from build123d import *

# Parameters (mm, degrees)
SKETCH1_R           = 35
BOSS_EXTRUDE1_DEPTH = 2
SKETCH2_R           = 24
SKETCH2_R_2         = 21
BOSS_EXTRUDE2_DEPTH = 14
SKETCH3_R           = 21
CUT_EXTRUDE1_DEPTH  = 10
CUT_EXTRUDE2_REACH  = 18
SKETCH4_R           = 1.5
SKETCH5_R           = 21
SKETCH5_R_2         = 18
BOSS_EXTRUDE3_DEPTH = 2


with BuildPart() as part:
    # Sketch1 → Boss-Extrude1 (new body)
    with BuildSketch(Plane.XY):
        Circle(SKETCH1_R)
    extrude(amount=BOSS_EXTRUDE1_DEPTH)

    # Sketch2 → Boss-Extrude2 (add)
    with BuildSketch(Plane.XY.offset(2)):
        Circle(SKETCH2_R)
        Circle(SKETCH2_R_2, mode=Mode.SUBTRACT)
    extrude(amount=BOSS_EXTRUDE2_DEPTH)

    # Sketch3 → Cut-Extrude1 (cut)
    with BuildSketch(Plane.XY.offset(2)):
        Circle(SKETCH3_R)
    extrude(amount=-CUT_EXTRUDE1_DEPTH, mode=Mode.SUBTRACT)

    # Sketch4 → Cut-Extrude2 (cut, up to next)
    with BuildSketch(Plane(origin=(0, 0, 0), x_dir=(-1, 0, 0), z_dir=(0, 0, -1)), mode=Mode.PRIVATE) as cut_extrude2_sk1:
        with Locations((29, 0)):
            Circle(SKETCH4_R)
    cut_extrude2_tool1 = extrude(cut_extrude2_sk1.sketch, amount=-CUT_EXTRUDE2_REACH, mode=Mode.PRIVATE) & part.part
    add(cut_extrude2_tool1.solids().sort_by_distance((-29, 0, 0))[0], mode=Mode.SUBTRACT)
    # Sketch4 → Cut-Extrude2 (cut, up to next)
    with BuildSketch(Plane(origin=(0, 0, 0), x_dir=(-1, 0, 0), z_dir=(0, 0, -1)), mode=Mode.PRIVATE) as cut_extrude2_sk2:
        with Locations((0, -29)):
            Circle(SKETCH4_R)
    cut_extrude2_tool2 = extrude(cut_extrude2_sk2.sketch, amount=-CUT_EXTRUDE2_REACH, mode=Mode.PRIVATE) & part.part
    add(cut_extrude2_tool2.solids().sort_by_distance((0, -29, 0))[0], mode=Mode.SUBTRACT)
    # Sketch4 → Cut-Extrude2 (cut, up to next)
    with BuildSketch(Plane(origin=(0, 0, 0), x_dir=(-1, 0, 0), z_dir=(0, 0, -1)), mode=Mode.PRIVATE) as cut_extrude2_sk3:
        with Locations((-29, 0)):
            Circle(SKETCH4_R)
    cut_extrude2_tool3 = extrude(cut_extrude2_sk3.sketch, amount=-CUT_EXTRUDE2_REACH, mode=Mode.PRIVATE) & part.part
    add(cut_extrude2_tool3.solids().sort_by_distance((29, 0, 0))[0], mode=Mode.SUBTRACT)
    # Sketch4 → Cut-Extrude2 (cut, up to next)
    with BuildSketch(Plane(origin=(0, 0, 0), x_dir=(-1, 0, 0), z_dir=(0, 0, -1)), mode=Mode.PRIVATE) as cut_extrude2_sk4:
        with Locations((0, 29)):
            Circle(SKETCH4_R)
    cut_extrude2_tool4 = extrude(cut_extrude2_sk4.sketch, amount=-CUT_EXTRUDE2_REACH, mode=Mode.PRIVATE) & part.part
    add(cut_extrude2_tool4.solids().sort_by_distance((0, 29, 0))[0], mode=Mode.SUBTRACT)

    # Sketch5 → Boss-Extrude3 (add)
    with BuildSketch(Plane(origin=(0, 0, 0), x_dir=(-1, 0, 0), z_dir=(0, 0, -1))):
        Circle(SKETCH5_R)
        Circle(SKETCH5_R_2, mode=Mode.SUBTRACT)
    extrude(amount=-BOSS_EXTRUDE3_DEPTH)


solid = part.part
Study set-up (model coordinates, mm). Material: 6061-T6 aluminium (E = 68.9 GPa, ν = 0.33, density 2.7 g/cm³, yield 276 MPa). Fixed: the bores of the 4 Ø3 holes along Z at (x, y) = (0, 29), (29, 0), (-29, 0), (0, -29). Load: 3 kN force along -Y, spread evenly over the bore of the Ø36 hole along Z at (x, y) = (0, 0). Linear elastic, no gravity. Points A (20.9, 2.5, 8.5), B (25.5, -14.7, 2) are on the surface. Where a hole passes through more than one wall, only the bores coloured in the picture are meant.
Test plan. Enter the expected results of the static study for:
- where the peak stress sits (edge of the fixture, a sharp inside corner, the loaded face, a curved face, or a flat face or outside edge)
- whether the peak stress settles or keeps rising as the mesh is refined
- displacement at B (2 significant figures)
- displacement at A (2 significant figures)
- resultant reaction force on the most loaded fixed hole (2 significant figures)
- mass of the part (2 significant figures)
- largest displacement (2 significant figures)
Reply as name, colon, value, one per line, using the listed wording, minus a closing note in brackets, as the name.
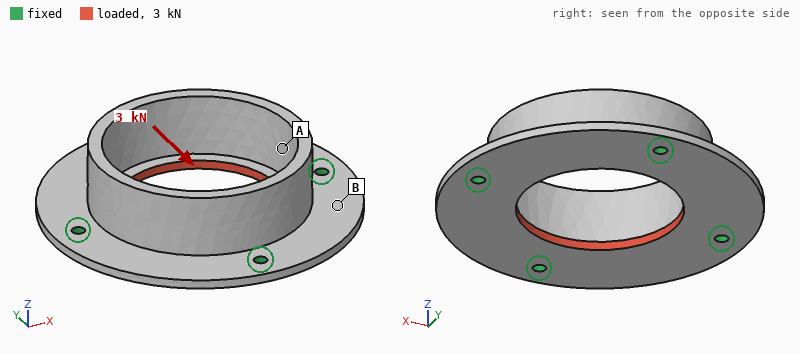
where the peak stress sits: edge of the fixture
whether the peak stress settles or keeps rising as the mesh is refined: keeps rising
displacement at B: 5.8 µm
displacement at A: 5.3 µm
resultant reaction force on the most loaded fixed hole: 790 N
mass of the part: 31 g
largest displacement: 8.9 µm
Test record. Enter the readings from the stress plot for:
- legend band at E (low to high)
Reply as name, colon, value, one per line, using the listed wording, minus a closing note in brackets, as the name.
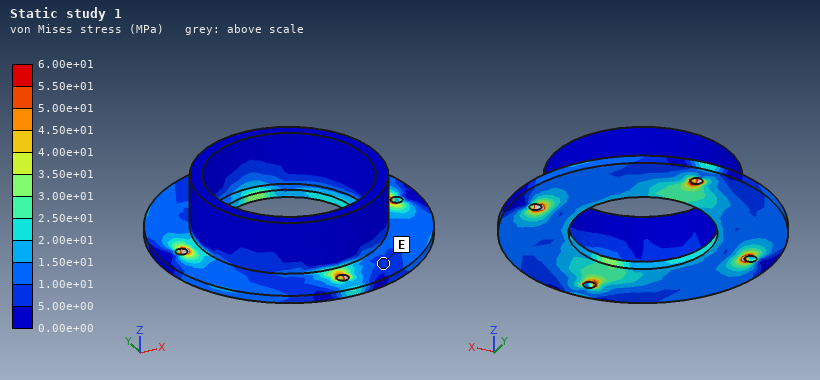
legend band at E: 5.00e+00 to 1.00e+01 MPa
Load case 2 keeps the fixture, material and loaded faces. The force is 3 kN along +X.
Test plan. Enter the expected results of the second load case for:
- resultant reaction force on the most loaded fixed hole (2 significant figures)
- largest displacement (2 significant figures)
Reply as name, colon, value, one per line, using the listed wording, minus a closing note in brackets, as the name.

resultant reaction force on the most loaded fixed hole: 790 N
largest displacement: 8.9 µm
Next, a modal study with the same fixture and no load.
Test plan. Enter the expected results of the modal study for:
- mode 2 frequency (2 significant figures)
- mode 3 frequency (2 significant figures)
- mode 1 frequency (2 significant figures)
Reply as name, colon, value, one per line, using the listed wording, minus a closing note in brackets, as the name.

mode 2 frequency: 7600 Hz
mode 3 frequency: 7600 Hz
mode 1 frequency: 5700 Hz
